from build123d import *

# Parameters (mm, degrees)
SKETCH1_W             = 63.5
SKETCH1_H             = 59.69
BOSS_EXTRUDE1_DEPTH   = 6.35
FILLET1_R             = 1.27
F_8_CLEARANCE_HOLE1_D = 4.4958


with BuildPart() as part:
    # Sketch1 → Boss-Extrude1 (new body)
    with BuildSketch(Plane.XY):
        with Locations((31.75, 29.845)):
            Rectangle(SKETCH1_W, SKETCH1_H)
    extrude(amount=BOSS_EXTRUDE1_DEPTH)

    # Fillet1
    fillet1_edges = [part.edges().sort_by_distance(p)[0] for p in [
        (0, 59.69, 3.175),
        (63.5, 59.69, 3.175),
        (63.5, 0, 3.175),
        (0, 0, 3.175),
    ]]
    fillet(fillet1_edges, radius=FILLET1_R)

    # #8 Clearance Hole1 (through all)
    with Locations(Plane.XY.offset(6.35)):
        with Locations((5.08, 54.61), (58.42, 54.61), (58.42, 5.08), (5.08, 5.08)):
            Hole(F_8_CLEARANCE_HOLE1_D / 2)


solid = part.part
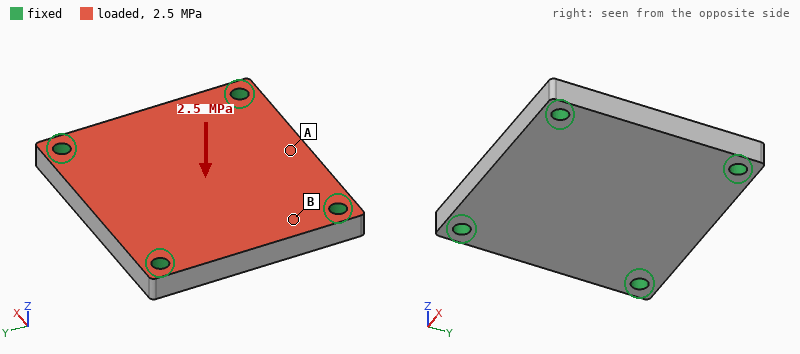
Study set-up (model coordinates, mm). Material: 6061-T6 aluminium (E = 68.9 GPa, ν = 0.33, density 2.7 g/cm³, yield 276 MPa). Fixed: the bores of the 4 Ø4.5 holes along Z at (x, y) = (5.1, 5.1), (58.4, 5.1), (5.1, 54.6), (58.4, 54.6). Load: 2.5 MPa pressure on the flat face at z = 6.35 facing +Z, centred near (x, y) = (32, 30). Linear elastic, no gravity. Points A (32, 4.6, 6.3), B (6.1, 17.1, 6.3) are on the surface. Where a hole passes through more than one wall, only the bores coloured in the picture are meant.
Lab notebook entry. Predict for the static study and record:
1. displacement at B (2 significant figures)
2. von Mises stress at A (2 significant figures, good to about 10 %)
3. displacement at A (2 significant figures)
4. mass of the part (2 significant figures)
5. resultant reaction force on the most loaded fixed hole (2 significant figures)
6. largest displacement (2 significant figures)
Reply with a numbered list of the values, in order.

1. 29 µm
2. 56 MPa
3. 56 µm
4. 64 g
5. 2.3 kN
6. 89 µm
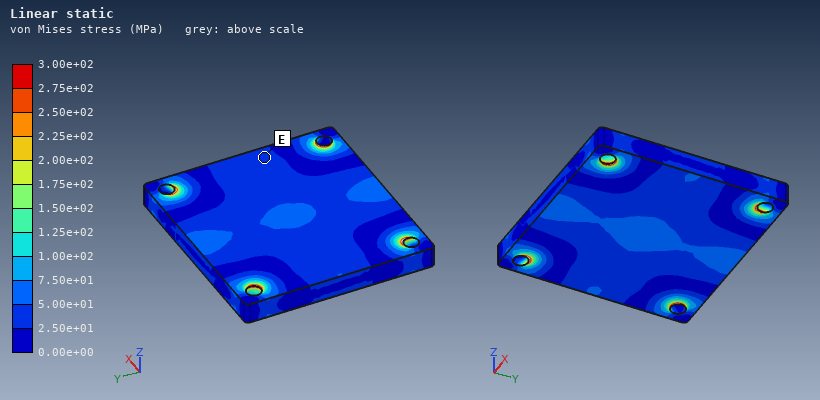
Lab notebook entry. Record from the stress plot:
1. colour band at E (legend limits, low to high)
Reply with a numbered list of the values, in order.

1. 2.50e+01 to 5.00e+01 MPa
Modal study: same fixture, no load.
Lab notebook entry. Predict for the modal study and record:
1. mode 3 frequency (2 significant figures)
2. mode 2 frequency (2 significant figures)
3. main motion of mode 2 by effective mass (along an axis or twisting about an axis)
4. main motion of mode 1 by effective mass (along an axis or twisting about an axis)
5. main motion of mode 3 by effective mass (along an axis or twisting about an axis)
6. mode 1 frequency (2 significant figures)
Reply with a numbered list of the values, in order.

1. 13 kHz
2. 12 kHz
3. twisting about X
4. along Z
5. twisting about Y
6. 7700 Hz
